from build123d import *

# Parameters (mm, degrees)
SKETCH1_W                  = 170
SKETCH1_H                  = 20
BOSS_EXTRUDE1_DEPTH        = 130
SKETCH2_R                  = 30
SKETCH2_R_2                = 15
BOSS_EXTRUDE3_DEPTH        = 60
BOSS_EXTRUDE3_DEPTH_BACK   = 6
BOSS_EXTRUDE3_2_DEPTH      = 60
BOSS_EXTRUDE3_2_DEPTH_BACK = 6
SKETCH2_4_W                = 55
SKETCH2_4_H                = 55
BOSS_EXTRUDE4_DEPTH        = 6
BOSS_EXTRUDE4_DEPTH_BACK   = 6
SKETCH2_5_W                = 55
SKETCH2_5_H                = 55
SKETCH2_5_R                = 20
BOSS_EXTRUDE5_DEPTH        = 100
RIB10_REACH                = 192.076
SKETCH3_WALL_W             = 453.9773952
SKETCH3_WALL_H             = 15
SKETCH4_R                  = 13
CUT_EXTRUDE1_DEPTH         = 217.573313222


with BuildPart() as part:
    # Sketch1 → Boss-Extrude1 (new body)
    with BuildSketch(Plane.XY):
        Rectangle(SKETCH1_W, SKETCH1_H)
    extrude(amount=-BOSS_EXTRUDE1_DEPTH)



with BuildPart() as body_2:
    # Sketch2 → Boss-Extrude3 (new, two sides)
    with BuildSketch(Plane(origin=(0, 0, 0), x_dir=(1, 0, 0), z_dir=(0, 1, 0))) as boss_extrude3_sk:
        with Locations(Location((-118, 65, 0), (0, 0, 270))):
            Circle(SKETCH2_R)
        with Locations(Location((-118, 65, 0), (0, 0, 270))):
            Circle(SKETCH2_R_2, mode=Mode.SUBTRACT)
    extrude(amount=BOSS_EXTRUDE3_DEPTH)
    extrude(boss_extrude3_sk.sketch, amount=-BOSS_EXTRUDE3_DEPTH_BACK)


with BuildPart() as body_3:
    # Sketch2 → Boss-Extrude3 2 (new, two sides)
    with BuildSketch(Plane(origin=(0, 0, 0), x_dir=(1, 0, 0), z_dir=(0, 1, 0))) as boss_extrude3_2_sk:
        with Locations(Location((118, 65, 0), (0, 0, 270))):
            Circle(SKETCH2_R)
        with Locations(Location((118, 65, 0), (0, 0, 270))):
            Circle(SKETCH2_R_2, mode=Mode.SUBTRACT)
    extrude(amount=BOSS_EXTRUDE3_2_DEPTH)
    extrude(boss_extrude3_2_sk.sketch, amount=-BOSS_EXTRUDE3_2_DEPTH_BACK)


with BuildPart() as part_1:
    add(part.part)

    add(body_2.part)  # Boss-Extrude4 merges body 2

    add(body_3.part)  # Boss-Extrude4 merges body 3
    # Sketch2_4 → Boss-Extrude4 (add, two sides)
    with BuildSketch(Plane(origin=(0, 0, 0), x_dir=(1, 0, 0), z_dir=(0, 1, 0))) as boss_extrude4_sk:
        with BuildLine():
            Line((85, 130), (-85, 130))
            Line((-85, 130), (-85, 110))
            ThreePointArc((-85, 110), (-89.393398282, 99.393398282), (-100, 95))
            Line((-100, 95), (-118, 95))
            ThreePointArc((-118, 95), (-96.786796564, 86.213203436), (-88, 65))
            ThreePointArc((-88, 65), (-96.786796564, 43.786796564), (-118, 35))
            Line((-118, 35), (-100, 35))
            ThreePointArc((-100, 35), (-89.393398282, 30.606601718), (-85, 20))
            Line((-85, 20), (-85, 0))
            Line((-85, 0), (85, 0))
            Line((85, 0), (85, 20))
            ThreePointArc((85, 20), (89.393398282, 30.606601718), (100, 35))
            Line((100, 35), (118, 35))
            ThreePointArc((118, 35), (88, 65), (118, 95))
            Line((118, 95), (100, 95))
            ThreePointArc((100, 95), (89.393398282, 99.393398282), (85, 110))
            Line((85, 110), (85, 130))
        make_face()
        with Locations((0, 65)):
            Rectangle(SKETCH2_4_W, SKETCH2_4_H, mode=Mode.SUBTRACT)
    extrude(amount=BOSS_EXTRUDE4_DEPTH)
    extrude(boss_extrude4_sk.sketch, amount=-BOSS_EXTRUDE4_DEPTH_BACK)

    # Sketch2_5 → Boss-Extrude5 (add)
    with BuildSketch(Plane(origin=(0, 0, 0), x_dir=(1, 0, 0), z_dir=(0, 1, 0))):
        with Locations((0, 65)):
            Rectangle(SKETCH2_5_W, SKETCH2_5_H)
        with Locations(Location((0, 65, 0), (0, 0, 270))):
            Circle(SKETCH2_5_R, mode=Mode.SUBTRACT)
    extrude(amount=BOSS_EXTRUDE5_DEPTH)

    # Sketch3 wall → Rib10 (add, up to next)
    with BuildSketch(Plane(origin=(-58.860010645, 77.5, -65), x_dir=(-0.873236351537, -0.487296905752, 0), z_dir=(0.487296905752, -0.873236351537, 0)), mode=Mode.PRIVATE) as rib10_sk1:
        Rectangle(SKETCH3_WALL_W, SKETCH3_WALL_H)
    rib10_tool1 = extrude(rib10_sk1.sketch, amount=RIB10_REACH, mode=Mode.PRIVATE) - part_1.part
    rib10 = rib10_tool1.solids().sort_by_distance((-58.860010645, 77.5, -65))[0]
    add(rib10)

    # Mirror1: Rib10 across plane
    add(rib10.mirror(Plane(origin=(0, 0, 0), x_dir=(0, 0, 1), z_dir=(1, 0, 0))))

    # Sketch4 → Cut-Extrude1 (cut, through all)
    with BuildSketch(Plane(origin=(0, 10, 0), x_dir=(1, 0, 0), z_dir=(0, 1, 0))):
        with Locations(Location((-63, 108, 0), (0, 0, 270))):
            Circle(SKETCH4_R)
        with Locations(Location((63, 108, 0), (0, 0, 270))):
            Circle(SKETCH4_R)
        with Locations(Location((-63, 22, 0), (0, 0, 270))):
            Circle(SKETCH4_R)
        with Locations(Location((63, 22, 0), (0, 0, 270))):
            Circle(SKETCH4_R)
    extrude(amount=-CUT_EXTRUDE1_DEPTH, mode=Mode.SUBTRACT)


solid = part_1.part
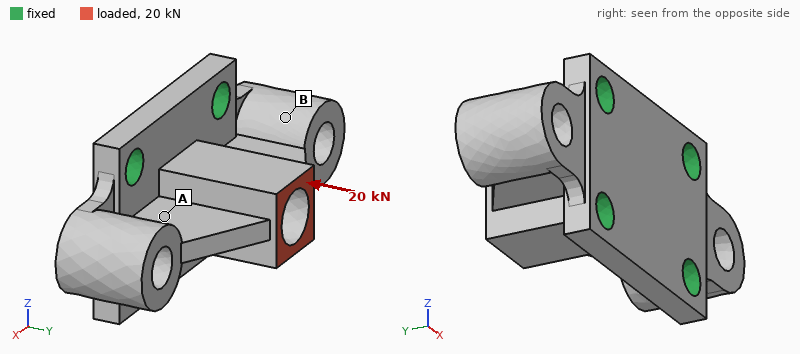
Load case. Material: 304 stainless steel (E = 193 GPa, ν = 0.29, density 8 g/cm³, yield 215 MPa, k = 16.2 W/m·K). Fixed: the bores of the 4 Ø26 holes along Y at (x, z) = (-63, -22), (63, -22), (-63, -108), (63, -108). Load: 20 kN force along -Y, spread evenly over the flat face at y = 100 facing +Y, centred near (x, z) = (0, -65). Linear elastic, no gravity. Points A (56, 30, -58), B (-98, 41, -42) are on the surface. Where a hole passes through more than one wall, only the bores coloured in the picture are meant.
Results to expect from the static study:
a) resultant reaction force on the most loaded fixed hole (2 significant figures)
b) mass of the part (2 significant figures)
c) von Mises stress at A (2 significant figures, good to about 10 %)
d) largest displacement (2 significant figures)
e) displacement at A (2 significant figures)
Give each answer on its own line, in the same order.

5.2 kN
7.8 kg
6.8 MPa
11 µm
3.3 µm
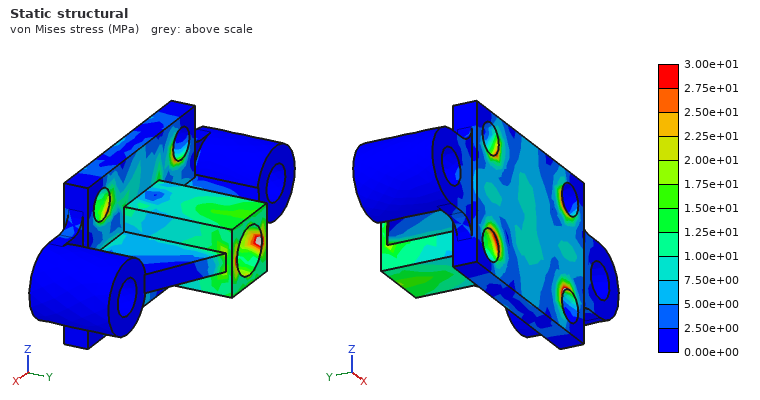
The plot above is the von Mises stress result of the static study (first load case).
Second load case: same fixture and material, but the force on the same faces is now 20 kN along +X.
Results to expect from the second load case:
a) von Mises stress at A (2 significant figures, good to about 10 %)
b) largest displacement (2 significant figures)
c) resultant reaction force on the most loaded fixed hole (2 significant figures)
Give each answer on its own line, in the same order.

17 MPa
31 µm
9.2 kN
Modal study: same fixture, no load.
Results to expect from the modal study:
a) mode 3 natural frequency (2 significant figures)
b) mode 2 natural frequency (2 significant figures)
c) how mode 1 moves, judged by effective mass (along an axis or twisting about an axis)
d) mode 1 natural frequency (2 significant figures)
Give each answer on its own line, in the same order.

2800 Hz
2700 Hz
along Z
2600 Hz
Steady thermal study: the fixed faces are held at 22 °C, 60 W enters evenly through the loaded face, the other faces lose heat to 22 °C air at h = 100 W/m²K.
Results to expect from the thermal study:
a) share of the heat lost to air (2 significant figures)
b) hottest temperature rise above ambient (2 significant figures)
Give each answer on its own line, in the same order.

96 %
57 K
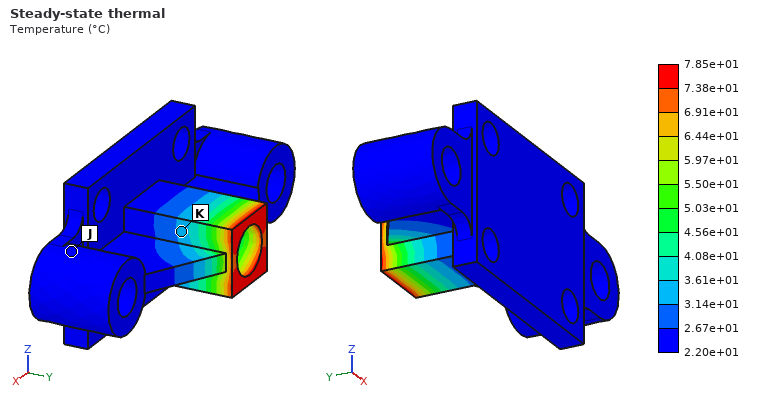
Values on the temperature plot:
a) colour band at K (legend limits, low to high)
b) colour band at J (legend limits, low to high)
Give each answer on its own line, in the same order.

3.14e+01 to 3.61e+01 °C
2.20e+01 to 2.67e+01 °C
